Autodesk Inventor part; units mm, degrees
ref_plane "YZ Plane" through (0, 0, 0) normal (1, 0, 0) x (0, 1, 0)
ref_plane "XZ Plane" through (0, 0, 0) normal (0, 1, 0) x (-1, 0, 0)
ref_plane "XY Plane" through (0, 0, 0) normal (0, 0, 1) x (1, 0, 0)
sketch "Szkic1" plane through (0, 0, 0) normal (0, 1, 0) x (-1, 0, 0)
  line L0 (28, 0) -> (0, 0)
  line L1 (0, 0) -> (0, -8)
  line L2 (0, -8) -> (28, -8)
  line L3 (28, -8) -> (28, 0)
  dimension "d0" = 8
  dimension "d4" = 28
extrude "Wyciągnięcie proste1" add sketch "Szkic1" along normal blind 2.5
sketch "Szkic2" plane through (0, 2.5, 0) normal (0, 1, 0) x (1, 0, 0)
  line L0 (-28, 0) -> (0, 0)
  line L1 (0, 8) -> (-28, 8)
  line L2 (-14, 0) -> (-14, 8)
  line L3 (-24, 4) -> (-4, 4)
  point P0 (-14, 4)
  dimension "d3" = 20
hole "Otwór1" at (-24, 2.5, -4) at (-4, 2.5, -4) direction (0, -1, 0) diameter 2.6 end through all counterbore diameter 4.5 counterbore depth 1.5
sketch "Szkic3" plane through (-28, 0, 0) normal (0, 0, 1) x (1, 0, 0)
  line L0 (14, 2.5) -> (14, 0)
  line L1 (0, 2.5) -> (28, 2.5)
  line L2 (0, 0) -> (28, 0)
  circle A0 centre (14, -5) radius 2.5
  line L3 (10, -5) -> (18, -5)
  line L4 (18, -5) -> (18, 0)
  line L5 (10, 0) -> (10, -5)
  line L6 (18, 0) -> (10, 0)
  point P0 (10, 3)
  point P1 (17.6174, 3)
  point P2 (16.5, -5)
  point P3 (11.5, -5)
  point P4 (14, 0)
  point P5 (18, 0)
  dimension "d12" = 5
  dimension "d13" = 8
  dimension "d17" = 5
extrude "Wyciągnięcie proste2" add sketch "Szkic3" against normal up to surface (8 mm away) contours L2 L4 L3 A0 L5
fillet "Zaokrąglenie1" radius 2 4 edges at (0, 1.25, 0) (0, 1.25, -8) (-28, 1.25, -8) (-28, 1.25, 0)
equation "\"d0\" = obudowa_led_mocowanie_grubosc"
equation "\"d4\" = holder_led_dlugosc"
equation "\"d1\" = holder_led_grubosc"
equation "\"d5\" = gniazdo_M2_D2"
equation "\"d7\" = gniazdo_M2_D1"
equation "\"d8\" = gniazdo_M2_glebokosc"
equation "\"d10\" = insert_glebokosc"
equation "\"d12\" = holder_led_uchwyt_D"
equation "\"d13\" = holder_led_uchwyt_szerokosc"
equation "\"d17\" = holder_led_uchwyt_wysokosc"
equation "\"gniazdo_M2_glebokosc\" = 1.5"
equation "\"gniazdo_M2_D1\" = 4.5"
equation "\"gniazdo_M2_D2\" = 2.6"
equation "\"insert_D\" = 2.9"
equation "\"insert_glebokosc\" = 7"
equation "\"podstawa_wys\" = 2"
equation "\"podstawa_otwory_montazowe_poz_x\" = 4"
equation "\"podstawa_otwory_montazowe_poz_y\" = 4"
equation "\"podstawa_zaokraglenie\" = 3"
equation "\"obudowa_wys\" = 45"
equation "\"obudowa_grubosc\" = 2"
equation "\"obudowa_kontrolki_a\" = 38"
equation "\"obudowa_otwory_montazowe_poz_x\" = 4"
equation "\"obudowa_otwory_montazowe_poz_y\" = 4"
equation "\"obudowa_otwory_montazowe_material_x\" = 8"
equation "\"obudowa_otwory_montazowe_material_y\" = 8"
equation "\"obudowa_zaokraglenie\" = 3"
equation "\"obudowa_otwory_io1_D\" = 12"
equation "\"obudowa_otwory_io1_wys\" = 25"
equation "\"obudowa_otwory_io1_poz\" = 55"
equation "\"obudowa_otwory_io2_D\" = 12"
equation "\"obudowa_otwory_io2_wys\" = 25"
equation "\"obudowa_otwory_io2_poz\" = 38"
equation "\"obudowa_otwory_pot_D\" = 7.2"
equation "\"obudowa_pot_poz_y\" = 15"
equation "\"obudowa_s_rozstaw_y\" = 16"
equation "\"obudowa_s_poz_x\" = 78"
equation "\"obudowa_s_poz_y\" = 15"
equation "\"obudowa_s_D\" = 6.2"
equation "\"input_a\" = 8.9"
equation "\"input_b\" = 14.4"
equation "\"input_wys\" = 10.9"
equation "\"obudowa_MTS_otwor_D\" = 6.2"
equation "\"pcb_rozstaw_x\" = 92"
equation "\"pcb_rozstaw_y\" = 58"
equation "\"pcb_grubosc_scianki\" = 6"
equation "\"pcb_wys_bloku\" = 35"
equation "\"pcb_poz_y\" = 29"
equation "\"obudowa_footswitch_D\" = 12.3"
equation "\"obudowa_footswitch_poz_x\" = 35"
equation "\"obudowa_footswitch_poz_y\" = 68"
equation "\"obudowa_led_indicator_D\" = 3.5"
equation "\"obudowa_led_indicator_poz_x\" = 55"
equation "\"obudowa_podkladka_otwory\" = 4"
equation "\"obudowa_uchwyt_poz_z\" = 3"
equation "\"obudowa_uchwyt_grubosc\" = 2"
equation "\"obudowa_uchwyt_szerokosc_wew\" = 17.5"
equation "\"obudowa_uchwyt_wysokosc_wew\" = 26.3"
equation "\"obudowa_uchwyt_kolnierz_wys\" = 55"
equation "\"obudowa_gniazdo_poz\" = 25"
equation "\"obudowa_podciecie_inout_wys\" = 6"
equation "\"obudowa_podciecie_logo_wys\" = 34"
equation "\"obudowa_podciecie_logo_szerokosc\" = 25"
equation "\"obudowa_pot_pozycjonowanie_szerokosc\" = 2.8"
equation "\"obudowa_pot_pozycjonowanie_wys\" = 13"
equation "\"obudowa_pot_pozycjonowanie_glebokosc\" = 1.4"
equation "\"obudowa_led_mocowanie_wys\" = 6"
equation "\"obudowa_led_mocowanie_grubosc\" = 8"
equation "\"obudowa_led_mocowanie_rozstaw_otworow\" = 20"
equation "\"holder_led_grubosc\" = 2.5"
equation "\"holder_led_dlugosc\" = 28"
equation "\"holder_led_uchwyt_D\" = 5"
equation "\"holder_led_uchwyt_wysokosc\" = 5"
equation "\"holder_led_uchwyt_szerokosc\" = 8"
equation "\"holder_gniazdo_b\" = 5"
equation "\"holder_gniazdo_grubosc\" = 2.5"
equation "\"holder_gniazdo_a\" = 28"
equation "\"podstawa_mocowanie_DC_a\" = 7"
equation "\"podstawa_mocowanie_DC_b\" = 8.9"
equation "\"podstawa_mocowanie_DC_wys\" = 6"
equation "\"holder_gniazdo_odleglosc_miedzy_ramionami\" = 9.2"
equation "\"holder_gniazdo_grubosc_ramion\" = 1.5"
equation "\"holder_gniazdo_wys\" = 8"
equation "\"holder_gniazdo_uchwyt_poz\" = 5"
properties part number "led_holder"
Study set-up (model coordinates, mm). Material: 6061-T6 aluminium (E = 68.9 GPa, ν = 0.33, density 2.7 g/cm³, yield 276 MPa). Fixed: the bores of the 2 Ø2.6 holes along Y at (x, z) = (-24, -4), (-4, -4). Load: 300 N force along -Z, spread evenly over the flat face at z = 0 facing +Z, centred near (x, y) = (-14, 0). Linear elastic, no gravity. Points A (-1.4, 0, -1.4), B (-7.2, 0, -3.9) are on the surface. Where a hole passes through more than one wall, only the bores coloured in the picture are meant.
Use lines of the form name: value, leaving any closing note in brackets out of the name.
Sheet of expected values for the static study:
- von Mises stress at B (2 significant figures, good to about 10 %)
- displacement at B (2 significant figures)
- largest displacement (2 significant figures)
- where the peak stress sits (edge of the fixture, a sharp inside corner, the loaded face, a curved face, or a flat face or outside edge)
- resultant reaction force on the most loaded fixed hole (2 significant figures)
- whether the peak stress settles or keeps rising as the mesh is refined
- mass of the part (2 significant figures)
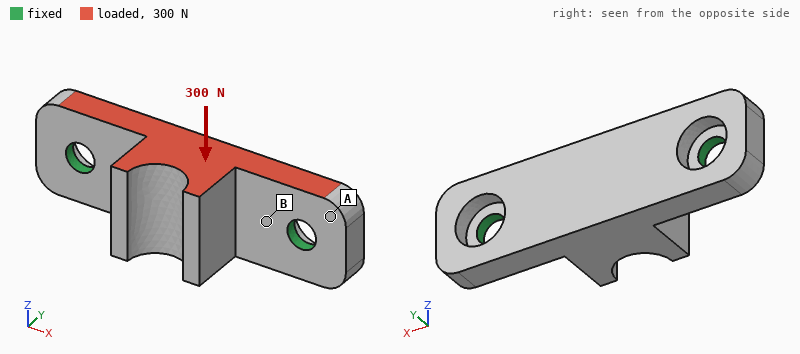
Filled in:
von Mises stress at B: 30 MPa
displacement at B: 2.4 µm
largest displacement: 11 µm
where the peak stress sits: edge of the fixture
resultant reaction force on the most loaded fixed hole: 150 N
whether the peak stress settles or keeps rising as the mesh is refined: keeps rising
mass of the part: 2.0 g
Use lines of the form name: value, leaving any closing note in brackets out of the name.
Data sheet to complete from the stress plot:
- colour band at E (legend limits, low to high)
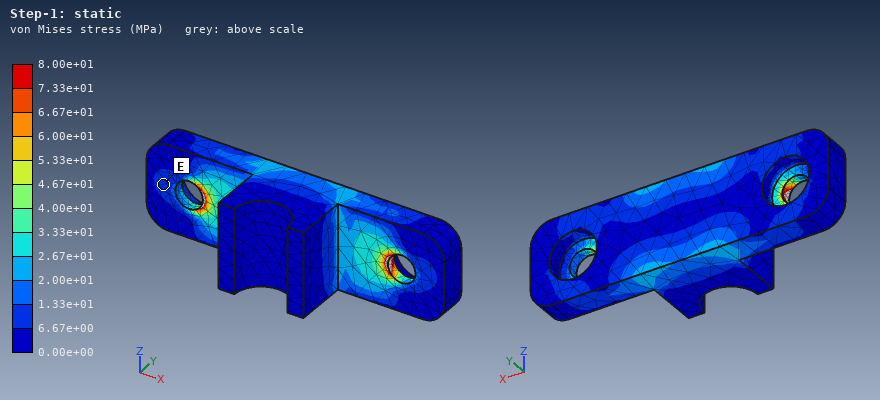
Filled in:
colour band at E: 6.67e+00 to 1.33e+01 MPa
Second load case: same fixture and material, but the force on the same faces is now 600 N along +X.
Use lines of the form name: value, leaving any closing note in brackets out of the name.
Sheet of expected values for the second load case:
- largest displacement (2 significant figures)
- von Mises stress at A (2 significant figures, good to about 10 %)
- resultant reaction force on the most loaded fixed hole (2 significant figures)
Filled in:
largest displacement: 11 µm
von Mises stress at A: 11 MPa
resultant reaction force on the most loaded fixed hole: 320 N
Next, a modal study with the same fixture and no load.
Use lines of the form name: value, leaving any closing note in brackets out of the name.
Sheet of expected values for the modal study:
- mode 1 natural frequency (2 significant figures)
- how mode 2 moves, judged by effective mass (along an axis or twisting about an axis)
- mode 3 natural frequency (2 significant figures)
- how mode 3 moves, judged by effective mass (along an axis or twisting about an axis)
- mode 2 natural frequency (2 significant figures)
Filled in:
mode 1 natural frequency: 17 kHz
how mode 2 moves, judged by effective mass: along Y
mode 3 natural frequency: 34 kHz
how mode 3 moves, judged by effective mass: along Z
mode 2 natural frequency: 20 kHz
